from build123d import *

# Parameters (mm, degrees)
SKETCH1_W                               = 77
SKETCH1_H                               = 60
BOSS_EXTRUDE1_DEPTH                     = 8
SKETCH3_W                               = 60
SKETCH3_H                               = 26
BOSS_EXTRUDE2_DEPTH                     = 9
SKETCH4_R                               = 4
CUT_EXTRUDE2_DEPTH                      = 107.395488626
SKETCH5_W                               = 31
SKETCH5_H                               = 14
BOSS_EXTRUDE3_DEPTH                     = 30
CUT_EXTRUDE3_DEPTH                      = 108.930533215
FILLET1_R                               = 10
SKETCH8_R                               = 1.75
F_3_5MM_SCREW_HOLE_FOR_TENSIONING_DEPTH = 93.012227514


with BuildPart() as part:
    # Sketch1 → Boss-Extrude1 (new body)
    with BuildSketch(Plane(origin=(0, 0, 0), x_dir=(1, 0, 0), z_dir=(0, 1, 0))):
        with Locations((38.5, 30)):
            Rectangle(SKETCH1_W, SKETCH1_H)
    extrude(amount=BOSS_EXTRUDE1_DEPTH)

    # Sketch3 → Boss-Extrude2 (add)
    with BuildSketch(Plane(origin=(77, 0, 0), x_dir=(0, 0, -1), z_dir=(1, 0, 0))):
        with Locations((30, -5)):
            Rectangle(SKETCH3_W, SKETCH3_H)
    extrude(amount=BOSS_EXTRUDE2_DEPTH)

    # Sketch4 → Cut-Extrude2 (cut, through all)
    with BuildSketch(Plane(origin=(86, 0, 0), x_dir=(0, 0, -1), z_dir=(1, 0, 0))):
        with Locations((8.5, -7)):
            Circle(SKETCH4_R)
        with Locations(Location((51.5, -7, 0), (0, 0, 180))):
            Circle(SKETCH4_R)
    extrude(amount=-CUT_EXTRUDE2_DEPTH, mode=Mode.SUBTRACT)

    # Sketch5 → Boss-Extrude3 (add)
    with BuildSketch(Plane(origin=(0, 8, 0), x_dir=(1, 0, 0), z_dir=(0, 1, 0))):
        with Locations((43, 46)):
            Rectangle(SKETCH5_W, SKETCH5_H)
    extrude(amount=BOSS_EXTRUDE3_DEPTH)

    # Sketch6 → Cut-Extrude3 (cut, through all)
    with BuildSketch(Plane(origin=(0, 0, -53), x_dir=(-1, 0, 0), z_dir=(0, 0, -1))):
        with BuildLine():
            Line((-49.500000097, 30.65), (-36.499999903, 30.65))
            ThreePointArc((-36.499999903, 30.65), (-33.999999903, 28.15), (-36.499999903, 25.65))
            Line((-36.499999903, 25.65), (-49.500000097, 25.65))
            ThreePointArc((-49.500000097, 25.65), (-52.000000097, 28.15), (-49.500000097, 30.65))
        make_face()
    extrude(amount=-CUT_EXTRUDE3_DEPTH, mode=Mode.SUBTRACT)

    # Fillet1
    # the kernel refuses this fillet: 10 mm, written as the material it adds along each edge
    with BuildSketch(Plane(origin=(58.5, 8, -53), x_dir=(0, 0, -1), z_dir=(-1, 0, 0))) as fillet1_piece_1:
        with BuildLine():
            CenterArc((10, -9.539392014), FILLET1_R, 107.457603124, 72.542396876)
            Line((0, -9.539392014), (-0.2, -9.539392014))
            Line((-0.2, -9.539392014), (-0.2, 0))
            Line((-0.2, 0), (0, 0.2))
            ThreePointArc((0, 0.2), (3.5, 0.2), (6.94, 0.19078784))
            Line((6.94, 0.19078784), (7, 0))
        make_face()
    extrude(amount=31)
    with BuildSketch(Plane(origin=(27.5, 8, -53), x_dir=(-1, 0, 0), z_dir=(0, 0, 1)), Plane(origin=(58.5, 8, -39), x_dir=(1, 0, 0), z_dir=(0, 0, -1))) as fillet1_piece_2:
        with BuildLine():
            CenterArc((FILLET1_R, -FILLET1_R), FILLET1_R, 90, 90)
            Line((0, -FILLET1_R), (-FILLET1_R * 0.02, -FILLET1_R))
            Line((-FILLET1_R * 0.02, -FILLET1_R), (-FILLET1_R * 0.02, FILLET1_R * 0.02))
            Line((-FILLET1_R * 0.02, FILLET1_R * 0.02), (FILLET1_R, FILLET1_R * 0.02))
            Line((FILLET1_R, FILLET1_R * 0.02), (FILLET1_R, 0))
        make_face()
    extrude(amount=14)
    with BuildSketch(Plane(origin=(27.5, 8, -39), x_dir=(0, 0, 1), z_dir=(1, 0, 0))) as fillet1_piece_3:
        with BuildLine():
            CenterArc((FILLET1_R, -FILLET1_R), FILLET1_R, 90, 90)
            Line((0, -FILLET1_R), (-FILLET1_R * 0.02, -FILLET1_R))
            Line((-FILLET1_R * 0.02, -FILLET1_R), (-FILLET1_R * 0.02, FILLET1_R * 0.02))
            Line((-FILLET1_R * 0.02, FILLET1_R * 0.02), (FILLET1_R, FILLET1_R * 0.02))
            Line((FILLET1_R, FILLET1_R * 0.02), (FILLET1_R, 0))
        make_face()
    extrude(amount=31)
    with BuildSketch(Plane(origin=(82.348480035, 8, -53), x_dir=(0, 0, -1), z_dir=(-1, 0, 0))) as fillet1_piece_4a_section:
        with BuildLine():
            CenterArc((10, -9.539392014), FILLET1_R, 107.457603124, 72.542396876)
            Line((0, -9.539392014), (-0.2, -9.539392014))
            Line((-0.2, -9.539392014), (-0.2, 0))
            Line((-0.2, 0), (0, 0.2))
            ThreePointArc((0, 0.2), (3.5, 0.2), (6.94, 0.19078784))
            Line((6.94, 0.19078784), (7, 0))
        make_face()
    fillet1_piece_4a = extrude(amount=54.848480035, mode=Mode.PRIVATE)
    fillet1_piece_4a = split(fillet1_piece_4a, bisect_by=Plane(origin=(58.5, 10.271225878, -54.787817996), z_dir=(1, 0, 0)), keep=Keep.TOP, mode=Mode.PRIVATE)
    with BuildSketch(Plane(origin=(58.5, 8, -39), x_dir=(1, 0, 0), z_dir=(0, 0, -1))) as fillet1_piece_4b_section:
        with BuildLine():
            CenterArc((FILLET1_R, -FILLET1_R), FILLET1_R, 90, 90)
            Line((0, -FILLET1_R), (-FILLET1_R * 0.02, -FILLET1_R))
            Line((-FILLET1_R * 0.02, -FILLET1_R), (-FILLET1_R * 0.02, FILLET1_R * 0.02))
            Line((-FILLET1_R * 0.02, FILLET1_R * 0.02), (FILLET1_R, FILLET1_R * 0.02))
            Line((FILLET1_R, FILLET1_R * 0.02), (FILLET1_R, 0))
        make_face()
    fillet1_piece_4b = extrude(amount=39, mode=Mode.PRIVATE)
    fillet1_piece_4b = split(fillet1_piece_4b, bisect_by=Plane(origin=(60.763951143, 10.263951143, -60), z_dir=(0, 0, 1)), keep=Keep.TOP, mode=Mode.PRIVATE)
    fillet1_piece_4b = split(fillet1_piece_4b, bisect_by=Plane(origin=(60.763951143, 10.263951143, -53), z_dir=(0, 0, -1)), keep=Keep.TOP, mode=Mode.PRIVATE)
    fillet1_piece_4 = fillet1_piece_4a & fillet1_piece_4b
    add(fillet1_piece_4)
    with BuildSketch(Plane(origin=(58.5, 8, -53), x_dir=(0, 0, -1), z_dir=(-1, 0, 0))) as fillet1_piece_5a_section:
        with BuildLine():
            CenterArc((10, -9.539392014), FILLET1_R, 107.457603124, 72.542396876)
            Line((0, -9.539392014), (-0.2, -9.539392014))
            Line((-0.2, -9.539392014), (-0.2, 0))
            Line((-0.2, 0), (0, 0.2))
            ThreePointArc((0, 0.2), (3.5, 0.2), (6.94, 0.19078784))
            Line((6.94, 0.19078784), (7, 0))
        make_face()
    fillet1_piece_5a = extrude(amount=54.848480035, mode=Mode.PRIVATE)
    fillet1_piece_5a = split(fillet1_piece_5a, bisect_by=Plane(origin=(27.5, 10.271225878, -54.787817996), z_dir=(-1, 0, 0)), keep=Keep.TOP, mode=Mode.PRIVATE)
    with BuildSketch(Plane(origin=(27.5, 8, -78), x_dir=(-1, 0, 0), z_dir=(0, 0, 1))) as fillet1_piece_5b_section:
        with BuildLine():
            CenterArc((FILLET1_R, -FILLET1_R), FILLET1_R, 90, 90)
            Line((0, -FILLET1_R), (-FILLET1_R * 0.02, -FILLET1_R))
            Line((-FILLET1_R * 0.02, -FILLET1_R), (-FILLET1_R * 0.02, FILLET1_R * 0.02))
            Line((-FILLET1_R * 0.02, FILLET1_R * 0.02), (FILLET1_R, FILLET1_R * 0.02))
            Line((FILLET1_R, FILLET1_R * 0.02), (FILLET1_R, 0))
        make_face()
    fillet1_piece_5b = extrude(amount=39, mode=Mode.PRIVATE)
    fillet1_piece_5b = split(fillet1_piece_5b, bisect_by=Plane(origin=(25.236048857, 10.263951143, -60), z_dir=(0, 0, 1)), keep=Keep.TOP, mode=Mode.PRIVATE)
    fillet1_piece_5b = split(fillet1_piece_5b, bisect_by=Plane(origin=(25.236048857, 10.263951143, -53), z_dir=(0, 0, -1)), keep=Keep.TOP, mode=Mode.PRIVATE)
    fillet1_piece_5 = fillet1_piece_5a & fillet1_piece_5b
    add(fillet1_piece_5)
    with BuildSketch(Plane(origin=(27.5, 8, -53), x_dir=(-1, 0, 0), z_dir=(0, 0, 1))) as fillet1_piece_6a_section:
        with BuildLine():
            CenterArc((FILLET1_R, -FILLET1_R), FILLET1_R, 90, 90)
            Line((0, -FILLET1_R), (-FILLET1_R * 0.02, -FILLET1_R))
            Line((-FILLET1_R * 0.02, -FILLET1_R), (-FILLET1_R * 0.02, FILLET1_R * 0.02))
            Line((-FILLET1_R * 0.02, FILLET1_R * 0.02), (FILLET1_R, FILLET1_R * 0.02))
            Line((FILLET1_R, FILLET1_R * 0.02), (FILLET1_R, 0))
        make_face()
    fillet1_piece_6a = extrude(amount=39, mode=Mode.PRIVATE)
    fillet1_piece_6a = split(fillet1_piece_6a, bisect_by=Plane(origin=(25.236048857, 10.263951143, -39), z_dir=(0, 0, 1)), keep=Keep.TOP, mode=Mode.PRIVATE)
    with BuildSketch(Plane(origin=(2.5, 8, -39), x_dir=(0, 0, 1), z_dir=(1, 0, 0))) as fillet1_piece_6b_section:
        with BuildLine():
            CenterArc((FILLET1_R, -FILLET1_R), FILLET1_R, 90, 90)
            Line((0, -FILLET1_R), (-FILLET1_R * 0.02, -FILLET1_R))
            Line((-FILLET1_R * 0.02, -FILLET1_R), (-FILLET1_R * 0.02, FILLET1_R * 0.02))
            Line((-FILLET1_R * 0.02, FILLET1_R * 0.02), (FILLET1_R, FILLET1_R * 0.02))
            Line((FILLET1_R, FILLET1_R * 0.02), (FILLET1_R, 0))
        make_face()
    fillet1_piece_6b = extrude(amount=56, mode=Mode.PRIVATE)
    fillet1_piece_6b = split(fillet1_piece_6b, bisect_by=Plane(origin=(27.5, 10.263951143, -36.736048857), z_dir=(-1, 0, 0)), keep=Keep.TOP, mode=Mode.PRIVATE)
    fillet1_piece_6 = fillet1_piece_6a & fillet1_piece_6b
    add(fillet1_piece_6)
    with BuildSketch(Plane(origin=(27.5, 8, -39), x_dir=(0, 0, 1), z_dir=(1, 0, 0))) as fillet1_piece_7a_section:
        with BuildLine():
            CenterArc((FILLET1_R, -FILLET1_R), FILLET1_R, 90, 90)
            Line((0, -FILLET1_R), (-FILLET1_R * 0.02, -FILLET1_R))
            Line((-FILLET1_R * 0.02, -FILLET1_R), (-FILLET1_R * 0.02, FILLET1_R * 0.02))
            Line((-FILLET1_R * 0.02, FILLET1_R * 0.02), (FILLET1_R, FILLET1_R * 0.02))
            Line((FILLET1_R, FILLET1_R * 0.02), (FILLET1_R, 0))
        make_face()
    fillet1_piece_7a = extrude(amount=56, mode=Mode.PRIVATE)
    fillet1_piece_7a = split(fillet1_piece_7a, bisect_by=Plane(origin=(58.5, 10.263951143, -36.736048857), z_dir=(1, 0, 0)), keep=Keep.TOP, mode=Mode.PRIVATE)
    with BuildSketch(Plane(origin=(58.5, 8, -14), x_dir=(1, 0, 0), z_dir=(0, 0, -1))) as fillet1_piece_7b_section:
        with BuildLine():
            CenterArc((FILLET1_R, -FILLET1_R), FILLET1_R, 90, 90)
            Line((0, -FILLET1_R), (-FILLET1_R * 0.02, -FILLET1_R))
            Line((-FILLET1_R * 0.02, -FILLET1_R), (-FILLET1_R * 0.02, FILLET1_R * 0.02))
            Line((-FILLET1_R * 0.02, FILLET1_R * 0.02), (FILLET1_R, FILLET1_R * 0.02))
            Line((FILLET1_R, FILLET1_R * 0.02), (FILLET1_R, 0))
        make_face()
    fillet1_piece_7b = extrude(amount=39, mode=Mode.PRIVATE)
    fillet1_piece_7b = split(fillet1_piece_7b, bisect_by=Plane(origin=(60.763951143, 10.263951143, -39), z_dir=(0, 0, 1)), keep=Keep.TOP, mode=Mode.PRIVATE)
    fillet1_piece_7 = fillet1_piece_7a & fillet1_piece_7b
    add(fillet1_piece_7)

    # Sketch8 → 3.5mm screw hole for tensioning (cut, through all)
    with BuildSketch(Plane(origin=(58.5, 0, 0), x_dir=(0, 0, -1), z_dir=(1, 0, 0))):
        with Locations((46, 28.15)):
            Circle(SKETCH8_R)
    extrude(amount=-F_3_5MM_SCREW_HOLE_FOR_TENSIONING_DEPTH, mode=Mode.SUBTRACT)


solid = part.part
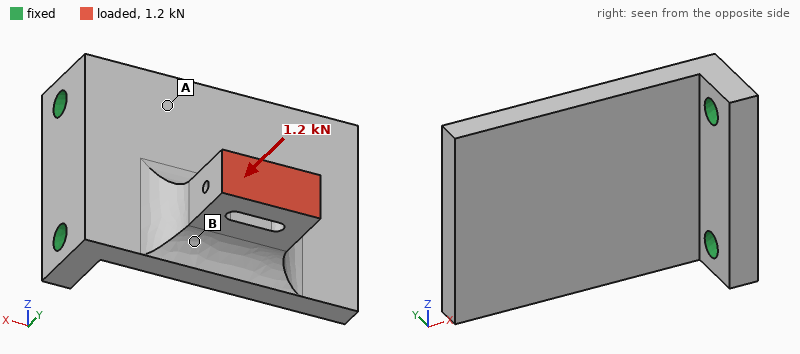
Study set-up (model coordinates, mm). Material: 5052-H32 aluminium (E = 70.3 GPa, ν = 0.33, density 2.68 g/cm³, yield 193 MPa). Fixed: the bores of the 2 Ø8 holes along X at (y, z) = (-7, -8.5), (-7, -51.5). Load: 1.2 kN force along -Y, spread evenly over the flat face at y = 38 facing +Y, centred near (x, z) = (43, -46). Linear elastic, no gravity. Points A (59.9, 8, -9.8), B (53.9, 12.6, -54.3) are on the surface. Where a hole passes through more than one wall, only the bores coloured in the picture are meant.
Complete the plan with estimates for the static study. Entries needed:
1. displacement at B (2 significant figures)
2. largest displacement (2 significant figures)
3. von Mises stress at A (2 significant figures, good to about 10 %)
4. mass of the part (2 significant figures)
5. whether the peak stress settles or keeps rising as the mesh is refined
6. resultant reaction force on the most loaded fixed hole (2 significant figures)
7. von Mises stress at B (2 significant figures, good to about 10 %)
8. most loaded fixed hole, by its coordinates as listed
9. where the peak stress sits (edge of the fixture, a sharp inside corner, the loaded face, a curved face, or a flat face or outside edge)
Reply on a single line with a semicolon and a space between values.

0.14 mm; 0.45 mm; 32 MPa; 170 g; keeps rising; 1.0 kN; 14 MPa; (-7, -51.5); edge of the fixture
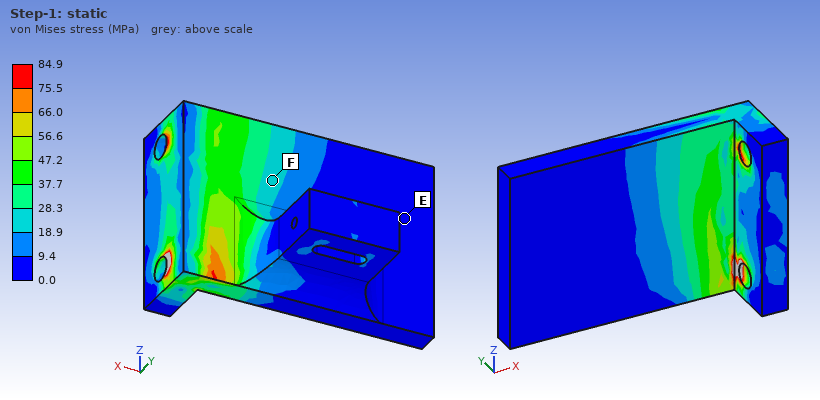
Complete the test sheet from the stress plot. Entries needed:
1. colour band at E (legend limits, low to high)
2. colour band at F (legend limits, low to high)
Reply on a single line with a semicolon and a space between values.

0.0 to 9.4 MPa; 18.9 to 28.3 MPa
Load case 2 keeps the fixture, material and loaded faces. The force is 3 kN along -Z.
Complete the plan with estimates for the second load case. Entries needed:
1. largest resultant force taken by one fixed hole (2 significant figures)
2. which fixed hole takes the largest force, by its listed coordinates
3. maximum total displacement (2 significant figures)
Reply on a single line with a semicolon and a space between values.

4.4 kN; (-7, -8.5); 0.33 mm
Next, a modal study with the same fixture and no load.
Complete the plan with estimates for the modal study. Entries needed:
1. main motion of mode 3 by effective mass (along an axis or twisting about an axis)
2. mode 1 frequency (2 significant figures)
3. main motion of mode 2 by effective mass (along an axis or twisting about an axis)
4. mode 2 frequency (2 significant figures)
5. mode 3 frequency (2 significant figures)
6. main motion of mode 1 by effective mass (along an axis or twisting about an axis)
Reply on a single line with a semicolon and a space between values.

along Z; 850 Hz; twisting about X; 2900 Hz; 3600 Hz; along Y
